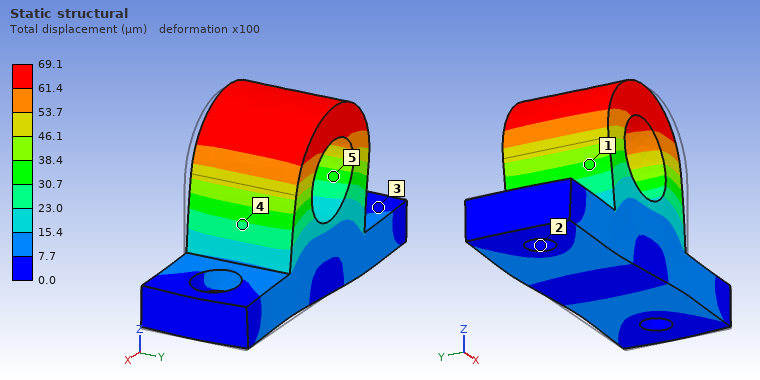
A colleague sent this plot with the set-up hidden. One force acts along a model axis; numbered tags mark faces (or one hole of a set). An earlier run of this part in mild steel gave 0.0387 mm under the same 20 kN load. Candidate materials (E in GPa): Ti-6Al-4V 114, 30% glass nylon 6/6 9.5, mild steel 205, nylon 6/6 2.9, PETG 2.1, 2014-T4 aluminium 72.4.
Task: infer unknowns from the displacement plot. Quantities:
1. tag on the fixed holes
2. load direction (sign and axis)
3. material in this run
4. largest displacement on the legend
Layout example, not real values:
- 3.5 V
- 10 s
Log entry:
- 2
- -X
- Ti-6Al-4V
- 69.1 µm
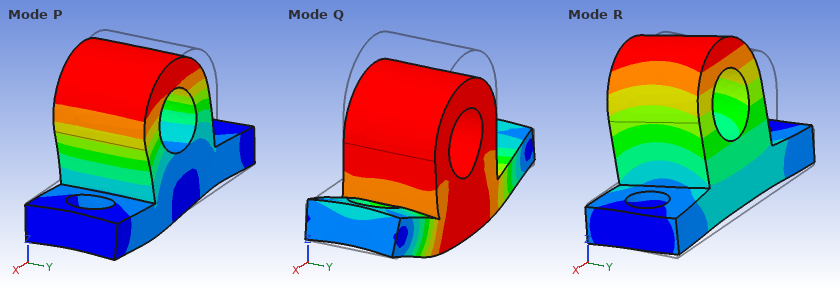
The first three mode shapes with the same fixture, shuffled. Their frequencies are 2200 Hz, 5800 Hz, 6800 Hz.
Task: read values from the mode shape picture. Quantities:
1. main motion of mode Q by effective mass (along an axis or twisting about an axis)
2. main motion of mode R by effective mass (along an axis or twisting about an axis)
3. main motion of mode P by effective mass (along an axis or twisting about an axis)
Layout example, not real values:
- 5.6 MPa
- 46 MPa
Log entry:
- along Z
- along Y
- along X
